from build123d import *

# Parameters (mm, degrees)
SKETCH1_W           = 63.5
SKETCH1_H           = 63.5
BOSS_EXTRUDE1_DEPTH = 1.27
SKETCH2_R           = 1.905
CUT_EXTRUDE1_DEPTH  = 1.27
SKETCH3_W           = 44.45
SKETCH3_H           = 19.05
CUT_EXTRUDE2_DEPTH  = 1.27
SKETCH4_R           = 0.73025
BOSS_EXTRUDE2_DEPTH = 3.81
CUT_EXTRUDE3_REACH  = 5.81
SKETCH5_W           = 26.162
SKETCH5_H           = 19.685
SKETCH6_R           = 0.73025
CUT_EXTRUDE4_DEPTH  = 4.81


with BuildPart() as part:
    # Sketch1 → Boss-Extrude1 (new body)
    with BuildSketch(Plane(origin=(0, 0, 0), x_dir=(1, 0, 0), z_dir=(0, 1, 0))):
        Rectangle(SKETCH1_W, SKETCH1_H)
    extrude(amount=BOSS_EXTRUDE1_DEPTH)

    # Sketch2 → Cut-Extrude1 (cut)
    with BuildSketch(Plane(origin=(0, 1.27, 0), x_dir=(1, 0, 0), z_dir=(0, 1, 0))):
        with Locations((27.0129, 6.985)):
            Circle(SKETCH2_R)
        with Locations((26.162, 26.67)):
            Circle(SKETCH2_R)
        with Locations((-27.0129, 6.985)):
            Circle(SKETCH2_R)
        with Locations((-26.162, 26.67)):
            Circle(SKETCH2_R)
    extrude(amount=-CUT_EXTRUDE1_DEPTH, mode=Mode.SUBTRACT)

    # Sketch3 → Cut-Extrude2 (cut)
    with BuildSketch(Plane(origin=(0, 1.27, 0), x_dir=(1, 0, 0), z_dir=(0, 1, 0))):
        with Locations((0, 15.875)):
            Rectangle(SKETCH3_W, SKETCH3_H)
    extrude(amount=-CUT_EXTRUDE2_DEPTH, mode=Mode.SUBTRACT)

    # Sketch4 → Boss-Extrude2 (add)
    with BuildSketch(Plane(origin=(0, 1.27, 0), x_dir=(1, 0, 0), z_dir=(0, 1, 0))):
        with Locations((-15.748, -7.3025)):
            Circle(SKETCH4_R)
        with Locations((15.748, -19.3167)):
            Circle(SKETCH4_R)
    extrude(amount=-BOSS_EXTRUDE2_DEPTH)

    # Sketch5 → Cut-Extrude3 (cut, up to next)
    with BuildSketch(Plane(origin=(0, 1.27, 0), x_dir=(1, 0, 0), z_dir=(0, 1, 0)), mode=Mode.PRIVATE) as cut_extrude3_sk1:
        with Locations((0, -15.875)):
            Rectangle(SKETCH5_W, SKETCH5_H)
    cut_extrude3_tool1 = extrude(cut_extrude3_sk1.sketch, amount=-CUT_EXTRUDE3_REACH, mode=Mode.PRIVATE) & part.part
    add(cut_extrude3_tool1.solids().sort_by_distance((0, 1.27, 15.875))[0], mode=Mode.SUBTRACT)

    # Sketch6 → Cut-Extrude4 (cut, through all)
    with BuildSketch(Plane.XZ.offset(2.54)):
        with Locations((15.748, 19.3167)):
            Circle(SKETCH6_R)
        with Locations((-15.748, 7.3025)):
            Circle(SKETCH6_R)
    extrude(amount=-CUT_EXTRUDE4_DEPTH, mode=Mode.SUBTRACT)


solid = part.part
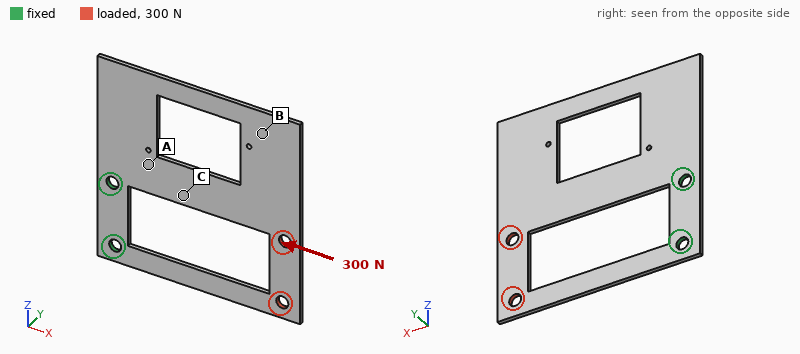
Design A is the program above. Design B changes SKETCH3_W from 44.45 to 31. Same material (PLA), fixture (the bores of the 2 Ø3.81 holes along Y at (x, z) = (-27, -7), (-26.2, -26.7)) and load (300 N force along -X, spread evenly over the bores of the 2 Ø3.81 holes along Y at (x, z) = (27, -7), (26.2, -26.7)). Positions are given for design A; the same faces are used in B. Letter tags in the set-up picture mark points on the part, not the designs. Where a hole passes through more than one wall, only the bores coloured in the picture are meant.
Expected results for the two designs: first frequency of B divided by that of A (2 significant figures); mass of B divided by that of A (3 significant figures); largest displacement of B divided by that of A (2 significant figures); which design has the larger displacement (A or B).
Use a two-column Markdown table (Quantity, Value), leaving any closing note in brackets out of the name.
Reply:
| Quantity | Value |
|---|---|
| first frequency of B divided by that of A | 1.1 |
| mass of B divided by that of A | 1.10 |
| largest displacement of B divided by that of A | 0.80 |
| which design has the larger displacement | A |
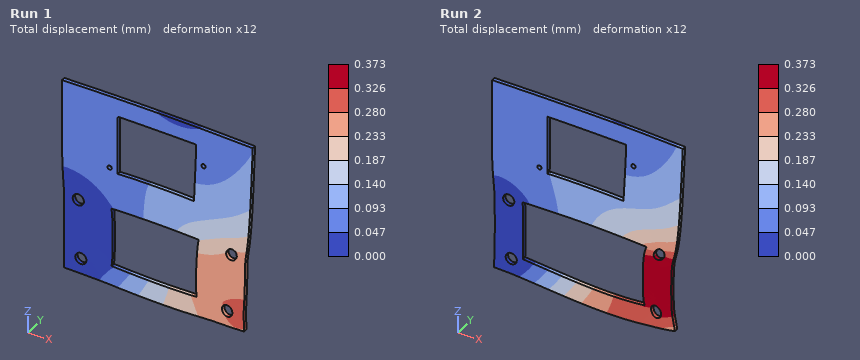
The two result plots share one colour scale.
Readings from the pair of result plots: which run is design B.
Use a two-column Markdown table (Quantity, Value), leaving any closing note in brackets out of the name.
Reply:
| Quantity | Value |
|---|---|
| which run is design B | Run 1 |
